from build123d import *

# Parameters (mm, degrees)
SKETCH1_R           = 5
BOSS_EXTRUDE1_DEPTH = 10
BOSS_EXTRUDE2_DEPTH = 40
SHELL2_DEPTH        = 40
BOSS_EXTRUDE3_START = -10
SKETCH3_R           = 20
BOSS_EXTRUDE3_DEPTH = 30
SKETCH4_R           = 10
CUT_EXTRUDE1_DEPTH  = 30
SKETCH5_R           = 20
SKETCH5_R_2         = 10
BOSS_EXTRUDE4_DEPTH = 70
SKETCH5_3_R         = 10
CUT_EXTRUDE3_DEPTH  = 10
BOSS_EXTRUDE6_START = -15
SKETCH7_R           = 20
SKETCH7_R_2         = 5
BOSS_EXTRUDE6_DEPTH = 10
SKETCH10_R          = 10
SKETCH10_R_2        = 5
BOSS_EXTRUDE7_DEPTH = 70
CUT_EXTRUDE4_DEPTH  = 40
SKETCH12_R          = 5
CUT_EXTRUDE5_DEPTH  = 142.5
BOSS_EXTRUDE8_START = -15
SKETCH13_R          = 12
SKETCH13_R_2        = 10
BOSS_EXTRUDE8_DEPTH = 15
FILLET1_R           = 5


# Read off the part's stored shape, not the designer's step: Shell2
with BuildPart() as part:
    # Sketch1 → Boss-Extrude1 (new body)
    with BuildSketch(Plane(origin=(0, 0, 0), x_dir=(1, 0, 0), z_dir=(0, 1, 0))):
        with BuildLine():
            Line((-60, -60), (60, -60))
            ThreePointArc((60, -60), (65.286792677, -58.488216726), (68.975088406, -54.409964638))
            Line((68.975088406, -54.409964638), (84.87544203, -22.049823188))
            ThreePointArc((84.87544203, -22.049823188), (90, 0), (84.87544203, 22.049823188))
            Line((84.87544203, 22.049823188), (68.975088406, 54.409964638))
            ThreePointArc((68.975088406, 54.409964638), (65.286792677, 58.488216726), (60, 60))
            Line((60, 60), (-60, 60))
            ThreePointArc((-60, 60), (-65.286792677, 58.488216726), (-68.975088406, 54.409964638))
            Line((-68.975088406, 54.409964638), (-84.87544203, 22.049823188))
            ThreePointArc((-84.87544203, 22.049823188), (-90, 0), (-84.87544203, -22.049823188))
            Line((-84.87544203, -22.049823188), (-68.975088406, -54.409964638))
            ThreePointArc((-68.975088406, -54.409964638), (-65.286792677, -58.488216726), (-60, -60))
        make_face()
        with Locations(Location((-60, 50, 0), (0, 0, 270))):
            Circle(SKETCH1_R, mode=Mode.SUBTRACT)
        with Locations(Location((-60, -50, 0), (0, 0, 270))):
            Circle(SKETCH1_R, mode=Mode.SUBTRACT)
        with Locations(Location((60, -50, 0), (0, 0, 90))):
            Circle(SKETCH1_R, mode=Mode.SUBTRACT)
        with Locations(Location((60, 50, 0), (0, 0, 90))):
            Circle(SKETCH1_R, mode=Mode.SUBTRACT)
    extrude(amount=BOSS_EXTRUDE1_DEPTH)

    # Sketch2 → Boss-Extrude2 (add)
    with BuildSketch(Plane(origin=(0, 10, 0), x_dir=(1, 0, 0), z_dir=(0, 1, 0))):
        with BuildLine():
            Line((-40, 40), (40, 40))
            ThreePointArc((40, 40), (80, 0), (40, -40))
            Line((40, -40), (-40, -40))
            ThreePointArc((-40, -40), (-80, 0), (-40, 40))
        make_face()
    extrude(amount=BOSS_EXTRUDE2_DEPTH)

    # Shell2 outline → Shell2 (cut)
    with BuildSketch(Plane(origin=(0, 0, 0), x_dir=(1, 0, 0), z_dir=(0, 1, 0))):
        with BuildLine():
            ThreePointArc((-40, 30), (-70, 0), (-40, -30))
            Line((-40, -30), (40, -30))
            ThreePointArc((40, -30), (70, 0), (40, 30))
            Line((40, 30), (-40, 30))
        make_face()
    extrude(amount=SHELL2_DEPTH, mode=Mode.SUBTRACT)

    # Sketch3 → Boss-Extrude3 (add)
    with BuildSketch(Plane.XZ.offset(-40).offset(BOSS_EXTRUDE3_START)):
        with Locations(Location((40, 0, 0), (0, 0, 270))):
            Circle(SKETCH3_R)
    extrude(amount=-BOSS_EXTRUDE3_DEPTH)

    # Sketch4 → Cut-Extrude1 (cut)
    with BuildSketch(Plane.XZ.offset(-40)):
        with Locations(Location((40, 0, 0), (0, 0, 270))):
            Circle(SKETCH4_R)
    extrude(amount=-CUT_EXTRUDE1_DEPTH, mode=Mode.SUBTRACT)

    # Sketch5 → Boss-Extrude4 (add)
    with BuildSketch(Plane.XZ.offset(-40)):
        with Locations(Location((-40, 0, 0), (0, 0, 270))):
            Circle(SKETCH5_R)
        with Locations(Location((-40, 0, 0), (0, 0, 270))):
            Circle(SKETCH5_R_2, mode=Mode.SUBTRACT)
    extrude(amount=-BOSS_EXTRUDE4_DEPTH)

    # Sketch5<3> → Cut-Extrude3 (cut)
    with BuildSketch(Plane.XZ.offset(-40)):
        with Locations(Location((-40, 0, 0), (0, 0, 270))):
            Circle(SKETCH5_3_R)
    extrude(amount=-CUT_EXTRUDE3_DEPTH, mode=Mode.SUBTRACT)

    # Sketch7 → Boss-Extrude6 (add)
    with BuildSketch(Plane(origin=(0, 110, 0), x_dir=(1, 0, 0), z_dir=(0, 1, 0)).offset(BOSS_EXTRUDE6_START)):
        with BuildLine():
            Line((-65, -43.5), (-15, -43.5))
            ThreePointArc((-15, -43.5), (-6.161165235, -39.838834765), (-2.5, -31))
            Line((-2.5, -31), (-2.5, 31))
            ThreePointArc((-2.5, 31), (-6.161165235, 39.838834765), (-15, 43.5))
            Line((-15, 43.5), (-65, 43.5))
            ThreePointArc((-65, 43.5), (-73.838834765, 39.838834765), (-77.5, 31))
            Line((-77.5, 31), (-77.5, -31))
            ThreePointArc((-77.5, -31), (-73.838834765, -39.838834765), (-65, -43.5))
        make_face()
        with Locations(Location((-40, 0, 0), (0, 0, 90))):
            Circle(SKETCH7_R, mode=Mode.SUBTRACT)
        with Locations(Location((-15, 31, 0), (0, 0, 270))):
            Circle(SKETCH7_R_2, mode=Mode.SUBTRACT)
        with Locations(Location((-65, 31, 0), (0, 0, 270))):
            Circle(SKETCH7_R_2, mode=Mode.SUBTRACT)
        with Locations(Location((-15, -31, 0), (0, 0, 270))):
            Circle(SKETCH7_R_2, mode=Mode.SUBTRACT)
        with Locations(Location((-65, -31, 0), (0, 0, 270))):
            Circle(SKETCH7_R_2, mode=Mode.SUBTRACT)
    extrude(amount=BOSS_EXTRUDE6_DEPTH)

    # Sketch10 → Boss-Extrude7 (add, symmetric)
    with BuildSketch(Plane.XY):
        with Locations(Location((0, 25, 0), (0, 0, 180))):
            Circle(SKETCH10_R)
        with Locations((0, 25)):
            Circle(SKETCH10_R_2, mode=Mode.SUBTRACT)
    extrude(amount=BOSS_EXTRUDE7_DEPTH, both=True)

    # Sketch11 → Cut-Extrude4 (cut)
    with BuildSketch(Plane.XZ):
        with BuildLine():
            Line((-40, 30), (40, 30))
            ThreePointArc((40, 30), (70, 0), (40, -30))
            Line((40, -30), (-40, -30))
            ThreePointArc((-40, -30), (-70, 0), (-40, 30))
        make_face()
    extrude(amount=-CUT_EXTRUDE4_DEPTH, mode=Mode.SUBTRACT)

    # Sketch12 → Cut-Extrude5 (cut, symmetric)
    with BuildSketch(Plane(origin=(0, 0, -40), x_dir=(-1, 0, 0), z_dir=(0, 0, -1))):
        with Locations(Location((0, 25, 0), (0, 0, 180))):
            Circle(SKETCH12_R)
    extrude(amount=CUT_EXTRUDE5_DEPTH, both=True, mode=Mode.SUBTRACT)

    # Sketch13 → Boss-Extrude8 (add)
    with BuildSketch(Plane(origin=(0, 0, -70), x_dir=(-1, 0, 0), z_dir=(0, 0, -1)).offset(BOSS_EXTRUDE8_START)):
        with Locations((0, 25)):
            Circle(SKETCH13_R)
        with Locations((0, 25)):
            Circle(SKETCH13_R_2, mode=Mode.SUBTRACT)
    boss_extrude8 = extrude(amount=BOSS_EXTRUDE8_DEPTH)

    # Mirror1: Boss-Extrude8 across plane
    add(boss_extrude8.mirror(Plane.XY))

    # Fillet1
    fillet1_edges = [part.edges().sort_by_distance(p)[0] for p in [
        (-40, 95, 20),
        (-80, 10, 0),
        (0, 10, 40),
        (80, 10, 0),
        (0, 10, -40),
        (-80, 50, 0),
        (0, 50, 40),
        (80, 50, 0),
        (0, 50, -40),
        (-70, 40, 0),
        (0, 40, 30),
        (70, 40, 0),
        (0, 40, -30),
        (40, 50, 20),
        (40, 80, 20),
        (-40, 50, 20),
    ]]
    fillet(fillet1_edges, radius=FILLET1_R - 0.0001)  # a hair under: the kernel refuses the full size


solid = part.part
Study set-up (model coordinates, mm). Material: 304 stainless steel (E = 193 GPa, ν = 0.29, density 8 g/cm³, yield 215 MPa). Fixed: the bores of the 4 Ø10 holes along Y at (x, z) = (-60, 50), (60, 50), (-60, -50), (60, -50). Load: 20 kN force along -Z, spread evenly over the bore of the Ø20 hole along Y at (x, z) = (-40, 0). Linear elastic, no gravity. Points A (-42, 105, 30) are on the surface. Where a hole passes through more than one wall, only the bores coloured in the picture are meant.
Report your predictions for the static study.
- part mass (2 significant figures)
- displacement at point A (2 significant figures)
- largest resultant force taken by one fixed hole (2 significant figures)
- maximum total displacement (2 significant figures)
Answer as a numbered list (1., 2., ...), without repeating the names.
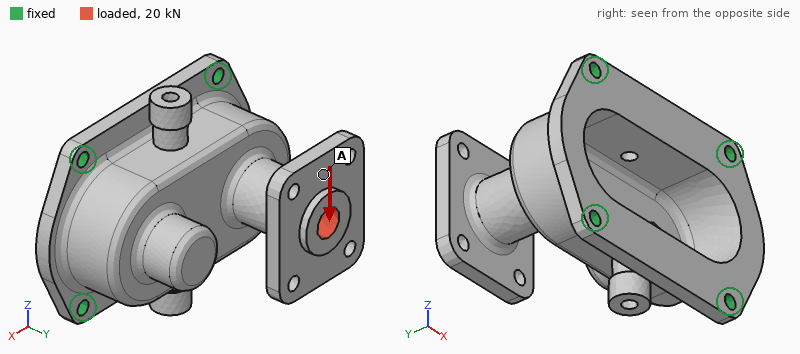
1. 3.9 kg
2. 0.11 mm
3. 12 kN
4. 0.12 mm
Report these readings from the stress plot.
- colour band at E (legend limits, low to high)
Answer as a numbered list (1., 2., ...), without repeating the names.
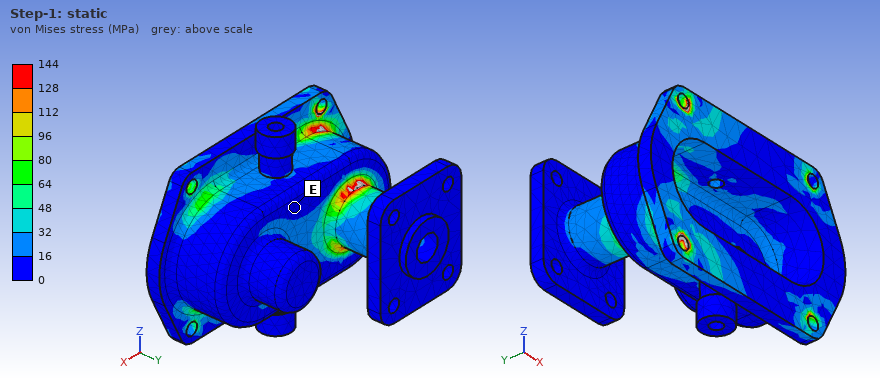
1. 0 to 16 MPa
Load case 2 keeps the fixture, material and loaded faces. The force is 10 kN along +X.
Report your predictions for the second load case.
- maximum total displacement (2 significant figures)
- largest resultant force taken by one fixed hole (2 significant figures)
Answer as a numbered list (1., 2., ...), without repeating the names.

1. 66 µm
2. 4.7 kN
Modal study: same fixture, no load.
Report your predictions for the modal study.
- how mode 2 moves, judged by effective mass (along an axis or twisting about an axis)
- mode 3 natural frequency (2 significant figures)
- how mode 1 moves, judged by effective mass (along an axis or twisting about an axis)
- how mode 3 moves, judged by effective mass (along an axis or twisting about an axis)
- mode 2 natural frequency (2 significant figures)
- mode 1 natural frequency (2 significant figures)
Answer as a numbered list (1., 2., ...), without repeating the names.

1. along Z
2. 3300 Hz
3. along X
4. along Y
5. 2000 Hz
6. 1900 Hz
